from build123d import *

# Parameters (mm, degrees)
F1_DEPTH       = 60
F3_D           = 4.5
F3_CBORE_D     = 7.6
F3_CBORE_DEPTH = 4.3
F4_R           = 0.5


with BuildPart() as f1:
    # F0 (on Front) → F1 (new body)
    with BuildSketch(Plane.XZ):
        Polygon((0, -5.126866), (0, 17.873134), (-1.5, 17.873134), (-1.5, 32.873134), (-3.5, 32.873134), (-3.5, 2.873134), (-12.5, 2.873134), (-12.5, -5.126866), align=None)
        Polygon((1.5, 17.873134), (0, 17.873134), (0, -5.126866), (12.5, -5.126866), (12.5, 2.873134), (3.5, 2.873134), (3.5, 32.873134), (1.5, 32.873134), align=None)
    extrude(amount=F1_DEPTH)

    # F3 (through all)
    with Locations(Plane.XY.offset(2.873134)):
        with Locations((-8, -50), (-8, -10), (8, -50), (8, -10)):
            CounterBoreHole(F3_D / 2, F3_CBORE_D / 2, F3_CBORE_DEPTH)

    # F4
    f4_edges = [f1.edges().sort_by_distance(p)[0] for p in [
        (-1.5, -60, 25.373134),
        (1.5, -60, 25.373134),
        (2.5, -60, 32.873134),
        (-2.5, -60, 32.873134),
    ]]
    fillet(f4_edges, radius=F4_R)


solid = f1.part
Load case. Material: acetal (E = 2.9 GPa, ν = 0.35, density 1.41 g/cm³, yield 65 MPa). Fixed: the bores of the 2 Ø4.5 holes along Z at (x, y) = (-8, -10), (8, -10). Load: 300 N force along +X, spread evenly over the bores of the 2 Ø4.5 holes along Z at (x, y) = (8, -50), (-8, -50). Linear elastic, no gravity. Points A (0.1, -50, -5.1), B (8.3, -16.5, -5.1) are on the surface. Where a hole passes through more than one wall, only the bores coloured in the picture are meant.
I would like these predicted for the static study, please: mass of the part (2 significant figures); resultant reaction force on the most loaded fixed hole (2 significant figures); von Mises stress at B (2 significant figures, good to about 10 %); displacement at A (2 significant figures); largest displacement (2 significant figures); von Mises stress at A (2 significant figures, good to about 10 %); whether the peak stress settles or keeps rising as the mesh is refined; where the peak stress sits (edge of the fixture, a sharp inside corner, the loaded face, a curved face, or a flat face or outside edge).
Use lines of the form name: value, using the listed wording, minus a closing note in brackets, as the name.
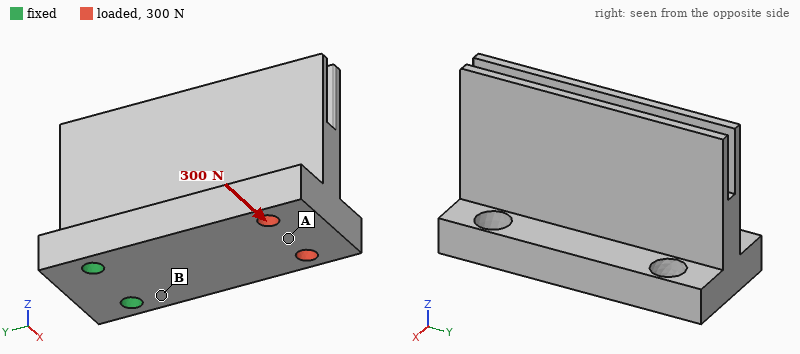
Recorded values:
mass of the part: 29 g
resultant reaction force on the most loaded fixed hole: 670 N
von Mises stress at B: 14 MPa
displacement at A: 0.37 mm
largest displacement: 0.50 mm
von Mises stress at A: 4.5 MPa
whether the peak stress settles or keeps rising as the mesh is refined: keeps rising
where the peak stress sits: edge of the fixture
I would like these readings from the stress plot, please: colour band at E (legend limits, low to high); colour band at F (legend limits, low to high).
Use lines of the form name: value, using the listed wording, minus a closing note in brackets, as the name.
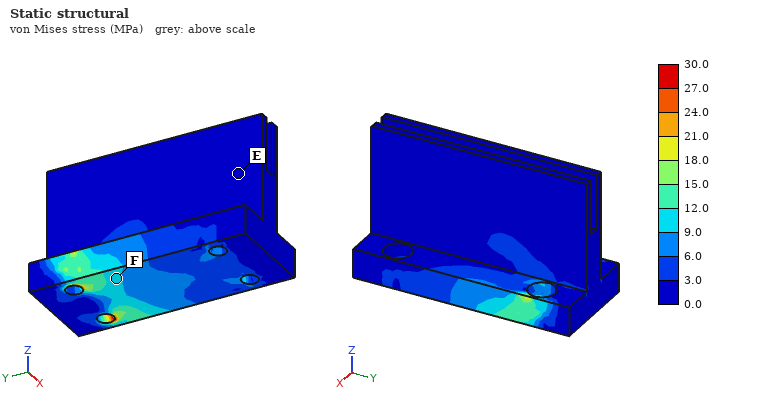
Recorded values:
colour band at E: 0.0 to 3.0 MPa
colour band at F: 9.0 to 12.0 MPa
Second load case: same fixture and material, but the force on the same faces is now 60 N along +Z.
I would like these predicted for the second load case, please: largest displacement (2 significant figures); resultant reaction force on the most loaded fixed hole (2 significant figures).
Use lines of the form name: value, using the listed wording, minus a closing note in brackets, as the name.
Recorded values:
largest displacement: 0.55 mm
resultant reaction force on the most loaded fixed hole: 33 N
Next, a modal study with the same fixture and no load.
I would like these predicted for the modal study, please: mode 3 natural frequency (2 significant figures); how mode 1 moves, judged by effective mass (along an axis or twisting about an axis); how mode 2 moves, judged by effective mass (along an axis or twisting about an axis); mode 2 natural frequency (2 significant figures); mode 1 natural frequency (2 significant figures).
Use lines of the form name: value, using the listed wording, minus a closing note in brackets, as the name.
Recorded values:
mode 3 natural frequency: 1500 Hz
how mode 1 moves, judged by effective mass: along Z
how mode 2 moves, judged by effective mass: along X
mode 2 natural frequency: 990 Hz
mode 1 natural frequency: 510 Hz
